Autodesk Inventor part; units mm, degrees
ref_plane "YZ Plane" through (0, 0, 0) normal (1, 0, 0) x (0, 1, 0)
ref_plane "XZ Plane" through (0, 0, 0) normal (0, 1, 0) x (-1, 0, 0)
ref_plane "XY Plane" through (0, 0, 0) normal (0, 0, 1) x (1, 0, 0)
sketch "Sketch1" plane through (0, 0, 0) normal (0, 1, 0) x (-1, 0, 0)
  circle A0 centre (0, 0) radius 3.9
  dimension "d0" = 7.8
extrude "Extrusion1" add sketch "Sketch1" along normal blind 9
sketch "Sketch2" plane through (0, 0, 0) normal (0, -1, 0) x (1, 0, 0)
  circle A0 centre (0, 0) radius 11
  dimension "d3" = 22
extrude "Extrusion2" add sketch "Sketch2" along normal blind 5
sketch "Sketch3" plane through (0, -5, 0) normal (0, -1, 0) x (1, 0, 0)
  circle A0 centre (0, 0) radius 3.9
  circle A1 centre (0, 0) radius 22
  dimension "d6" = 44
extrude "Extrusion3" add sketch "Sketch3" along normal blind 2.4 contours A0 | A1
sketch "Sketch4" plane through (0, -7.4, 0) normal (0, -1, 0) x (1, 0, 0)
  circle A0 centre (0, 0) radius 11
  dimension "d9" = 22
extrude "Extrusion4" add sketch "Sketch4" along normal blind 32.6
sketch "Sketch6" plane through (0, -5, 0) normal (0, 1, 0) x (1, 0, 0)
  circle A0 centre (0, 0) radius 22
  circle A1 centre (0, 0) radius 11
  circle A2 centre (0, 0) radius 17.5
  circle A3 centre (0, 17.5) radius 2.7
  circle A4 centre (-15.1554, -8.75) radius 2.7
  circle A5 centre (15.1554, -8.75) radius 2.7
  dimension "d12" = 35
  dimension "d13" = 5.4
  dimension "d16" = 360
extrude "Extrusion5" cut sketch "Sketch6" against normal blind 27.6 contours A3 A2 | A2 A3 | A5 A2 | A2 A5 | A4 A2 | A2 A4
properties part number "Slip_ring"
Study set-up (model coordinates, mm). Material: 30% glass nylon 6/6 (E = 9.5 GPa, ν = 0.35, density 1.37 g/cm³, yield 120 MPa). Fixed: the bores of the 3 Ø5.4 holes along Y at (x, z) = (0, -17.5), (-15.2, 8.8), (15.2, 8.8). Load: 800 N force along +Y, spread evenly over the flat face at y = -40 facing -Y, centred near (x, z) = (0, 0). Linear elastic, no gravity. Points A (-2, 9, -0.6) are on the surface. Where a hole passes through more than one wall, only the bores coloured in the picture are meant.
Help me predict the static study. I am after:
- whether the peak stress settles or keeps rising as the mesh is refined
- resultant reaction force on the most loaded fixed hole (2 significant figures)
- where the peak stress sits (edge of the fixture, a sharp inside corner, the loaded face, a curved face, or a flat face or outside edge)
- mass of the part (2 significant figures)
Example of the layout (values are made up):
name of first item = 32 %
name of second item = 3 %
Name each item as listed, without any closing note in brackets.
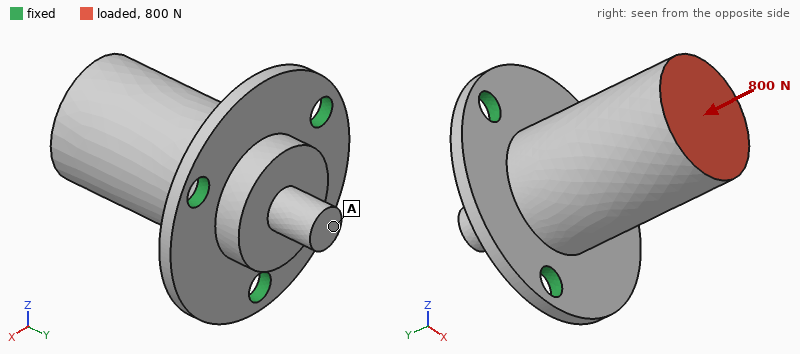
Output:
whether the peak stress settles or keeps rising as the mesh is refined = keeps rising
resultant reaction force on the most loaded fixed hole = 270 N
where the peak stress sits = edge of the fixture
mass of the part = 25 g
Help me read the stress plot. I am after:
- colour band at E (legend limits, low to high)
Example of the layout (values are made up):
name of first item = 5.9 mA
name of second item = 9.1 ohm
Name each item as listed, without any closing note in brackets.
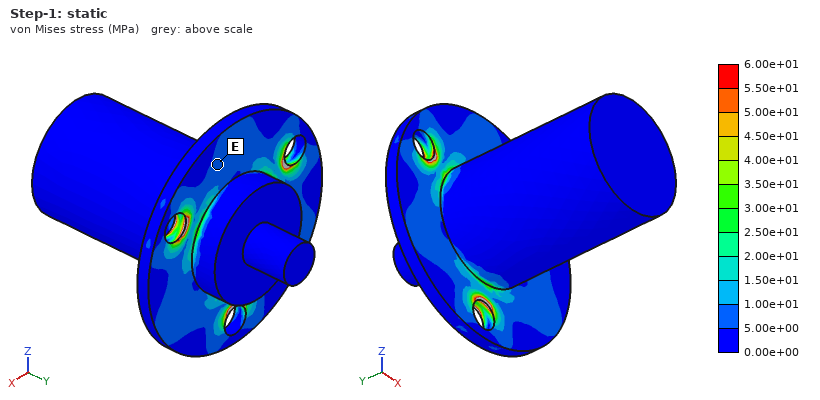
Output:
colour band at E = 5.00e+00 to 1.00e+01 MPa
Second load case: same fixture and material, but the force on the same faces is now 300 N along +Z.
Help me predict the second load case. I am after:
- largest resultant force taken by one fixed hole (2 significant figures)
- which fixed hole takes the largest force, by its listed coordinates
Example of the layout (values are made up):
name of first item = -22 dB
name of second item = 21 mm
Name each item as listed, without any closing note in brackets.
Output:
largest resultant force taken by one fixed hole = 480 N
which fixed hole takes the largest force, by its listed coordinates = (0, -17.5)
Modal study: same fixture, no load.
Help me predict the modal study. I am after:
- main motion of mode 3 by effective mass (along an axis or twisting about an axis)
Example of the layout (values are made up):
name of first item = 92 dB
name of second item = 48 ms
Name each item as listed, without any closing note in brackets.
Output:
main motion of mode 3 by effective mass = along Y
